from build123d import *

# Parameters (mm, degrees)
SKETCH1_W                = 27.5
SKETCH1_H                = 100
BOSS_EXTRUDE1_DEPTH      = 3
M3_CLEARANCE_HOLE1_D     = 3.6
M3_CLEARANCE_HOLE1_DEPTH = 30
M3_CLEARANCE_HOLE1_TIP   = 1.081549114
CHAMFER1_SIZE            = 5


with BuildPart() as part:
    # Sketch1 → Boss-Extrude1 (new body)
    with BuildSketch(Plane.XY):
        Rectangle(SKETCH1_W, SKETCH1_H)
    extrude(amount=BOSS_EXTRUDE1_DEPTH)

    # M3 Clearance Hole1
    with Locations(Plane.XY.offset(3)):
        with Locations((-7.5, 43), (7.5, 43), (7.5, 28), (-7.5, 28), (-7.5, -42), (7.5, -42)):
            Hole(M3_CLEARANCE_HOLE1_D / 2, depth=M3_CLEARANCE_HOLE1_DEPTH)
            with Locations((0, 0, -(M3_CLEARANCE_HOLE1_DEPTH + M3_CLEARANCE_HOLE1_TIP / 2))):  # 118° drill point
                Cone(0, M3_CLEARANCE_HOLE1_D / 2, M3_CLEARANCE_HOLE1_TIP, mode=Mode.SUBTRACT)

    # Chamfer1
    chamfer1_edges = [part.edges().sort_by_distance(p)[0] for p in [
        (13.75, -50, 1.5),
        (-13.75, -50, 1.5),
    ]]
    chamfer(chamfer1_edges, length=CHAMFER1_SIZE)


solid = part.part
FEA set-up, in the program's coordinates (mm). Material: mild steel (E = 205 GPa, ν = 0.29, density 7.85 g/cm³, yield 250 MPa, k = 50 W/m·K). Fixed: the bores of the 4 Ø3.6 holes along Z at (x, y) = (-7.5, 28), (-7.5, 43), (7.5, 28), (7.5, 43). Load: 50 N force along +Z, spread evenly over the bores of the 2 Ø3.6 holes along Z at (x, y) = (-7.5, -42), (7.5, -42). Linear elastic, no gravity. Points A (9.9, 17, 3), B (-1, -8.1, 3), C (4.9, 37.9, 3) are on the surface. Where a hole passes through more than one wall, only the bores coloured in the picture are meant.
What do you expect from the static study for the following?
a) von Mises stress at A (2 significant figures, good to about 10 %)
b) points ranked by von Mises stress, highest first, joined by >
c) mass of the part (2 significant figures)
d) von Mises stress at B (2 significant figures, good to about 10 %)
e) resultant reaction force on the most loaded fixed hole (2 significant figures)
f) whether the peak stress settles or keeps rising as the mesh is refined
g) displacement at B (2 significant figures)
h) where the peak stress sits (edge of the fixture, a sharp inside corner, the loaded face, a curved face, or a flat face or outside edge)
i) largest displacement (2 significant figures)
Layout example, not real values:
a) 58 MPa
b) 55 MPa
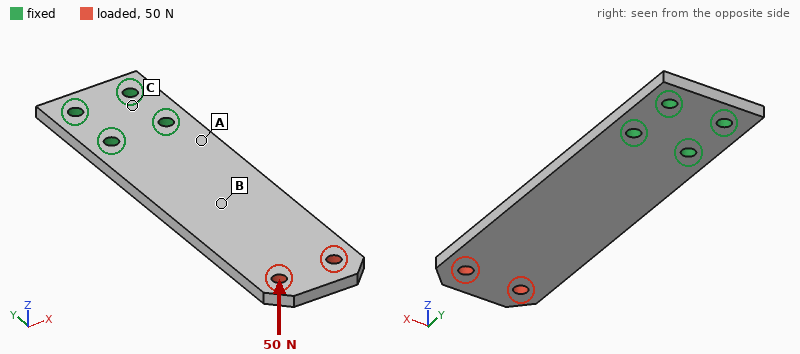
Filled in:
a) 70 MPa
b) A > B > C
c) 63 g
d) 41 MPa
e) 43 N
f) keeps rising
g) 0.14 mm
h) edge of the fixture
i) 0.51 mm
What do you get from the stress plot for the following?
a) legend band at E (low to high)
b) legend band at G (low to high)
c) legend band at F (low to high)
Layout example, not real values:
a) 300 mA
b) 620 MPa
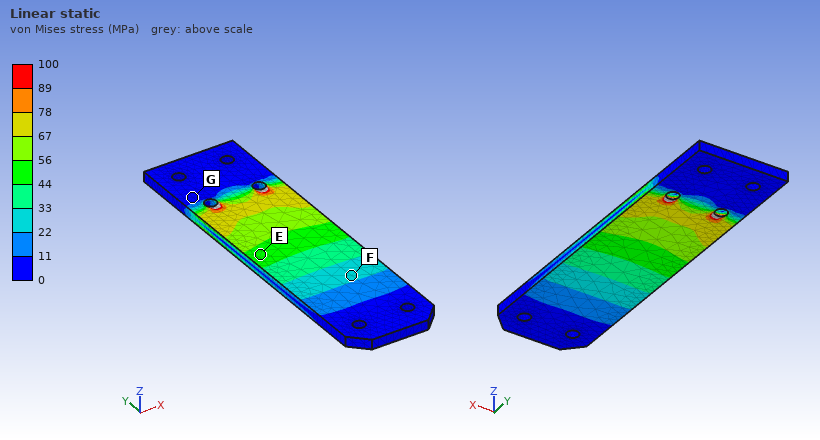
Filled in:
a) 44 to 56 MPa
b) 0 to 11 MPa
c) 22 to 33 MPa
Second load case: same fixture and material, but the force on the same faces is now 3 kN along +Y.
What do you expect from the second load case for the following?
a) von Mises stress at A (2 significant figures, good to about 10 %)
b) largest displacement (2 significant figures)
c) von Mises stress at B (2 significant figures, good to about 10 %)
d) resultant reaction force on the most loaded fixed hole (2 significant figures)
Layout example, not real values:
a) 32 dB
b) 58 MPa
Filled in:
a) 37 MPa
b) 14 µm
c) 36 MPa
d) 1.3 kN
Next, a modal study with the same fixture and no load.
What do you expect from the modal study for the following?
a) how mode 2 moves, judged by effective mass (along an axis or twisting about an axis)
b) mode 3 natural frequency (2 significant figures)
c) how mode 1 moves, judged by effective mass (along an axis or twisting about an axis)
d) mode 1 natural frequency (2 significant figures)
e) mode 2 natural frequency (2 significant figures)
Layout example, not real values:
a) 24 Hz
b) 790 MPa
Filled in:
a) twisting about Y
b) 2700 Hz
c) along Z
d) 430 Hz
e) 2400 Hz
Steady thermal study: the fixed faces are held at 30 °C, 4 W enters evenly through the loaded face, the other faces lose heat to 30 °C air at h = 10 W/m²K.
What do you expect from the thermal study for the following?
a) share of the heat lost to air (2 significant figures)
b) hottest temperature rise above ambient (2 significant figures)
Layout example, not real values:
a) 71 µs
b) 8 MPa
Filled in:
a) 32 %
b) 54 K
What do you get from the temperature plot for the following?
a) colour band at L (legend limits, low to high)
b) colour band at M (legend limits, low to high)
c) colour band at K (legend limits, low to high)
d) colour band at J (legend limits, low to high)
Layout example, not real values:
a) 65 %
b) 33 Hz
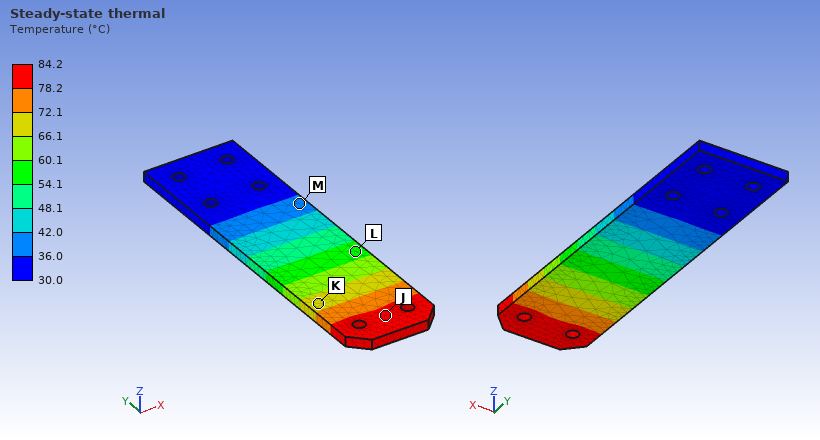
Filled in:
a) 54.1 to 60.1 °C
b) 36.0 to 42.0 °C
c) 66.1 to 72.1 °C
d) 78.2 to 84.2 °C
